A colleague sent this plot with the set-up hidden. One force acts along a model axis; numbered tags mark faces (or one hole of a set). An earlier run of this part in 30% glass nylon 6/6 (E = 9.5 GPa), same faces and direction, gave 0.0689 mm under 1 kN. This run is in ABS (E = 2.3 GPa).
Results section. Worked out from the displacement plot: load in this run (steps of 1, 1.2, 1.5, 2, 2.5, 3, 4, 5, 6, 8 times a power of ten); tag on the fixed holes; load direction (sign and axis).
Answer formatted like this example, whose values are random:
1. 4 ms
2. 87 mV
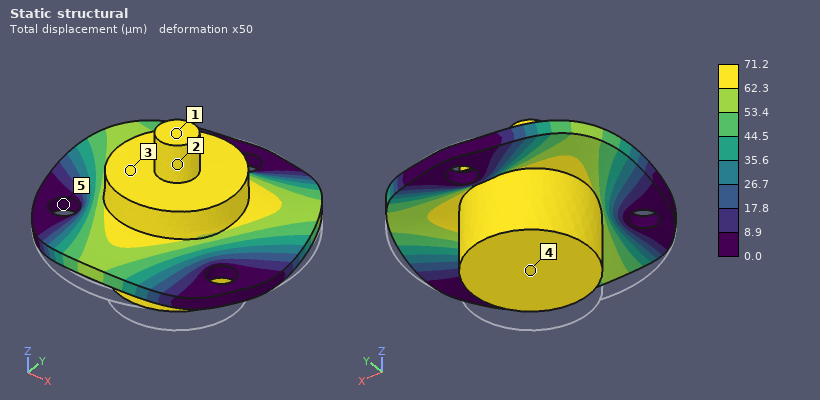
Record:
1. 250 N
2. 5
3. +Z
